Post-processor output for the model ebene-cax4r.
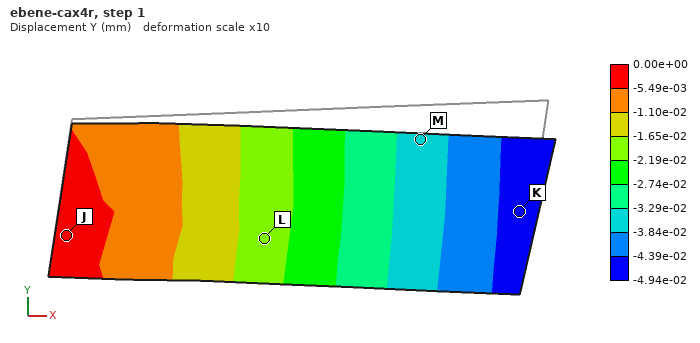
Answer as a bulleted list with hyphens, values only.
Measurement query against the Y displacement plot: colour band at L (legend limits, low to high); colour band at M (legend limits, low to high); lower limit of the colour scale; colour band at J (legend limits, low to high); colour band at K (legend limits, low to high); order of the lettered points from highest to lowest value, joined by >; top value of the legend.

- -2.19e-02 to -1.65e-02 mm
- -3.84e-02 to -3.29e-02 mm
- -4.94e-02 mm
- -5.49e-03 to 0.00e+00 mm
- -4.94e-02 to -4.39e-02 mm
- J > L > M > K
- 0.00e+00 mm
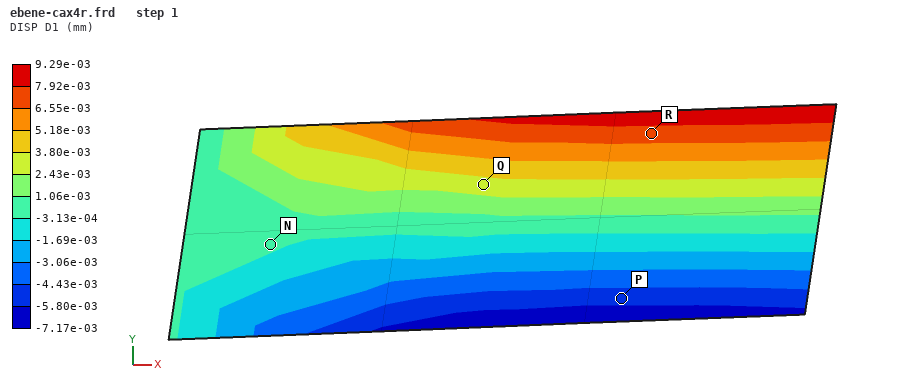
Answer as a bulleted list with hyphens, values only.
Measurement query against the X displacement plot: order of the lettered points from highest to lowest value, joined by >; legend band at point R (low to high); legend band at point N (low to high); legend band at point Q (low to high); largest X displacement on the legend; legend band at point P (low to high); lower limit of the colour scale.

- R > Q > N > P
- 6.55e-03 to 7.92e-03 mm
- -3.13e-04 to 1.06e-03 mm
- 2.43e-03 to 3.80e-03 mm
- 9.29e-03 mm
- -5.80e-03 to -4.43e-03 mm
- -7.17e-03 mm
